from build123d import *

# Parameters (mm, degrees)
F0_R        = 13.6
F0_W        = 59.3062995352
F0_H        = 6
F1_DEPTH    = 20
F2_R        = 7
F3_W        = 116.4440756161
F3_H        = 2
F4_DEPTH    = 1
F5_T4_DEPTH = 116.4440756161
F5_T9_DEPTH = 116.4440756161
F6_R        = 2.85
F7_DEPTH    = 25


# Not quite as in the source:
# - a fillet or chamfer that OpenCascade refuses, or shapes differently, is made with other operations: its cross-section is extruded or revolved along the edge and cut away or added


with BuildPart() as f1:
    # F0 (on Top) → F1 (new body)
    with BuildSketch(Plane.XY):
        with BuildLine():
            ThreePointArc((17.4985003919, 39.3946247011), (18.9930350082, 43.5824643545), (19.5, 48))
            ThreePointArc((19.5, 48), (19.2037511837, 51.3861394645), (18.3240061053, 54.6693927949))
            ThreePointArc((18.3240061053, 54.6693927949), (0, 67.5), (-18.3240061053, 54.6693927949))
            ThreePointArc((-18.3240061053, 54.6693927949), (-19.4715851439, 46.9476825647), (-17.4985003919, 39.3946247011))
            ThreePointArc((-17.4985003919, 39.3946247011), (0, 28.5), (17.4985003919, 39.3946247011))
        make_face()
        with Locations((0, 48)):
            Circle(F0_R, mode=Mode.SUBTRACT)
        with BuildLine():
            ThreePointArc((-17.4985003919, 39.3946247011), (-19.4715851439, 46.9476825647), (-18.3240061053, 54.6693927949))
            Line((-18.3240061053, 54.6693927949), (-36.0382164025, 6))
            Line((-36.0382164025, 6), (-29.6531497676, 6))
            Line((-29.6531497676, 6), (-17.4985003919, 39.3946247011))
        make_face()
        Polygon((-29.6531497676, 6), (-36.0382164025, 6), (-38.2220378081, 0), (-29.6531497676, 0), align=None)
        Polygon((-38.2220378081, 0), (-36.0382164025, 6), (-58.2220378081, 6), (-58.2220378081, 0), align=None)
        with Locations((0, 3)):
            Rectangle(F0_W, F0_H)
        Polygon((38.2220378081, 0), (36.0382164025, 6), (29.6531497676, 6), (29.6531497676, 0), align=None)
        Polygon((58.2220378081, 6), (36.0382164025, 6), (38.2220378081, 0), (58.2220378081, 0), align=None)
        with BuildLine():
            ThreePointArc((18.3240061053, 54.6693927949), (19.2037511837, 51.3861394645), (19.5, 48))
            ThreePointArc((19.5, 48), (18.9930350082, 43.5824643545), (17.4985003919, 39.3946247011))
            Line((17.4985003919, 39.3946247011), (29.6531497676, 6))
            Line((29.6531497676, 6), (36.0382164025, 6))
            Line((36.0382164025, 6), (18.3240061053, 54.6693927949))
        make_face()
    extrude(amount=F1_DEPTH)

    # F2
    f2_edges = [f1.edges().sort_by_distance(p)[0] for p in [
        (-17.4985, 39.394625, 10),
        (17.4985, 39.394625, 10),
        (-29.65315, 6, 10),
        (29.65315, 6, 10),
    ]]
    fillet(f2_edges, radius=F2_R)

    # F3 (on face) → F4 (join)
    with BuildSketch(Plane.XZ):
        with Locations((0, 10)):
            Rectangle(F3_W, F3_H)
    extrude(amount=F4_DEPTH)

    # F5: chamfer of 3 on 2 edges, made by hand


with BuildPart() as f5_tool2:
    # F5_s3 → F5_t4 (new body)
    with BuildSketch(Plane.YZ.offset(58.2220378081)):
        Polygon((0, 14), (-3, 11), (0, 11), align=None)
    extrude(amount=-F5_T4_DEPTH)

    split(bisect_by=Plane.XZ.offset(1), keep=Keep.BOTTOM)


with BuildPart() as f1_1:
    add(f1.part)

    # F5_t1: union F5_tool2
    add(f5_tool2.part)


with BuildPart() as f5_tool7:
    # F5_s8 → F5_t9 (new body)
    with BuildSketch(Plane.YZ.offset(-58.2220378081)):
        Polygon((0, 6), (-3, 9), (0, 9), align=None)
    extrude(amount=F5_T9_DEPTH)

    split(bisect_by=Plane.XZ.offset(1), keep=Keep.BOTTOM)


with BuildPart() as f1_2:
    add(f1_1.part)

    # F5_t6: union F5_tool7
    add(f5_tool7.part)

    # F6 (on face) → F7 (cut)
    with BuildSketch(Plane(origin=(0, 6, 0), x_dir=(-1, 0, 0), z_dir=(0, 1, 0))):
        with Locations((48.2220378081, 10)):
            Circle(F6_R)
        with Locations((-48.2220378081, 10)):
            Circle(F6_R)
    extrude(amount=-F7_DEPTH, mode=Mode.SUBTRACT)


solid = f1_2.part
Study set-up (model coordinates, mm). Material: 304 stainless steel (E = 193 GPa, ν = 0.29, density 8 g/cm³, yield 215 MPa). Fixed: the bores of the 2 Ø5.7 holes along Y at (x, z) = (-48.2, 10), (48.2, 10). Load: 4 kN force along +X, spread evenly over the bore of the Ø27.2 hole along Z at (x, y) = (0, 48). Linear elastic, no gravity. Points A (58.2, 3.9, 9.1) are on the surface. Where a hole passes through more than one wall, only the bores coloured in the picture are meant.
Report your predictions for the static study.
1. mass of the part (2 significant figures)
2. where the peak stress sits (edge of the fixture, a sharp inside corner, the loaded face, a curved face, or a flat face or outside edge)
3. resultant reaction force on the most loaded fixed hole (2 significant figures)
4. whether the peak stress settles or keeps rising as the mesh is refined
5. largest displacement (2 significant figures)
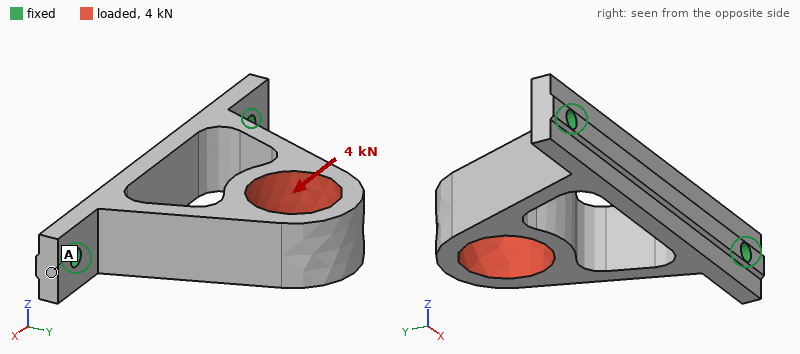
310 g
edge of the fixture
2.9 kN
keeps rising
60 µm
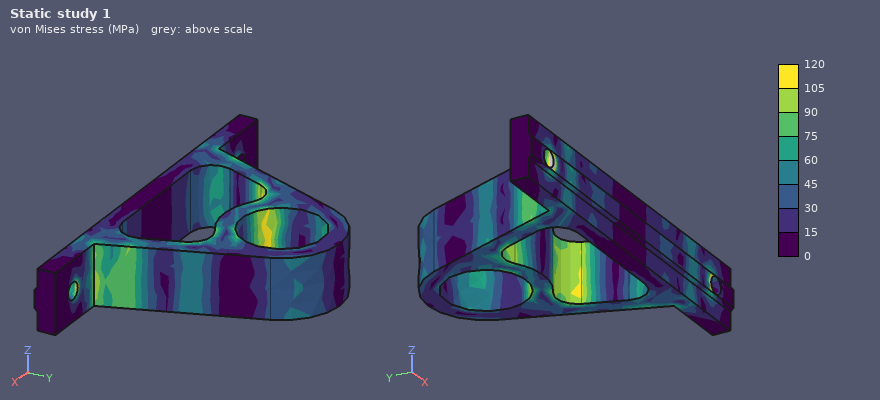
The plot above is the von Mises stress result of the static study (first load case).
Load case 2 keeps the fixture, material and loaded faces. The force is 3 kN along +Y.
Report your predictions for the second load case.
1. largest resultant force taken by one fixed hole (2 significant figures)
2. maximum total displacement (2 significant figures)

1.7 kN
16 µm
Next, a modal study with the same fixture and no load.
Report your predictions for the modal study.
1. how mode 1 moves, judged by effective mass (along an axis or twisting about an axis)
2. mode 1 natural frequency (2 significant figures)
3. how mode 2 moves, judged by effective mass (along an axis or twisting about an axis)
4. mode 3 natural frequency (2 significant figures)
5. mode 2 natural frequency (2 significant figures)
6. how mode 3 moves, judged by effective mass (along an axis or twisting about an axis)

along Z
1200 Hz
along X
4300 Hz
3500 Hz
along Y
